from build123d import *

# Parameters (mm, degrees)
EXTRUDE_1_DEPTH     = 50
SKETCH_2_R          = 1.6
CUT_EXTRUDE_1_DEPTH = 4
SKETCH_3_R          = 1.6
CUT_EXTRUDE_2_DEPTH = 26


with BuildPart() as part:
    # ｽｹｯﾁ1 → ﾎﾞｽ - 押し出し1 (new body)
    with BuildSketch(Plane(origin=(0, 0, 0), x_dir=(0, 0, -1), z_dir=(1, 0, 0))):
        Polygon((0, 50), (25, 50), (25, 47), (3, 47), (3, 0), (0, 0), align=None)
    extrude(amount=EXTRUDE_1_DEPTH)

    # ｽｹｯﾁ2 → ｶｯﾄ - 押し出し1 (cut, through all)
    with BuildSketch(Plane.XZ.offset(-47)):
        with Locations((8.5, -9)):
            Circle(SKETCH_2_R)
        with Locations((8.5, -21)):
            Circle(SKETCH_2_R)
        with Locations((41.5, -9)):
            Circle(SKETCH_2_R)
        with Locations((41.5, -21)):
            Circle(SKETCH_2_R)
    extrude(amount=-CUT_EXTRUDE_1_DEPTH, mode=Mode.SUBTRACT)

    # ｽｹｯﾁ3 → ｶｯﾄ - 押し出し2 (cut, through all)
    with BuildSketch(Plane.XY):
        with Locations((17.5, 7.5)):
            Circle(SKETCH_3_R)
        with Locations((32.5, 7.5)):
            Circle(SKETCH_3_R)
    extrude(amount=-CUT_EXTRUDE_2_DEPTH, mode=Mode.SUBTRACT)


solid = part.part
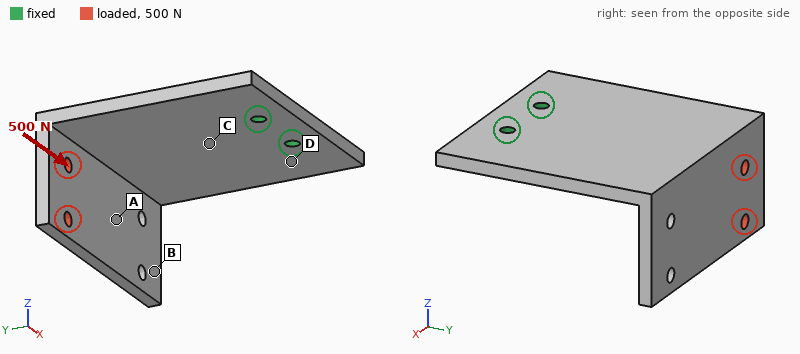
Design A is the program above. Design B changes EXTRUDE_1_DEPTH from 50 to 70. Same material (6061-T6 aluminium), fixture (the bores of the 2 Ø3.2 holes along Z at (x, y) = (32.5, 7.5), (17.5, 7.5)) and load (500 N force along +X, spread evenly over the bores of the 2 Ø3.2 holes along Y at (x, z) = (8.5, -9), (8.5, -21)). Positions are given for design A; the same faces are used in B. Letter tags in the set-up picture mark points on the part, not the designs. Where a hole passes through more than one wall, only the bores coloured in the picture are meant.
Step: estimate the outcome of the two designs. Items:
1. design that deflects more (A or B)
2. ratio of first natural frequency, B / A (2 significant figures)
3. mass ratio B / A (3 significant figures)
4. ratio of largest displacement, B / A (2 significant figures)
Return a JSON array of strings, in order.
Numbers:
["B", "0.85", "1.41", "1.2"]
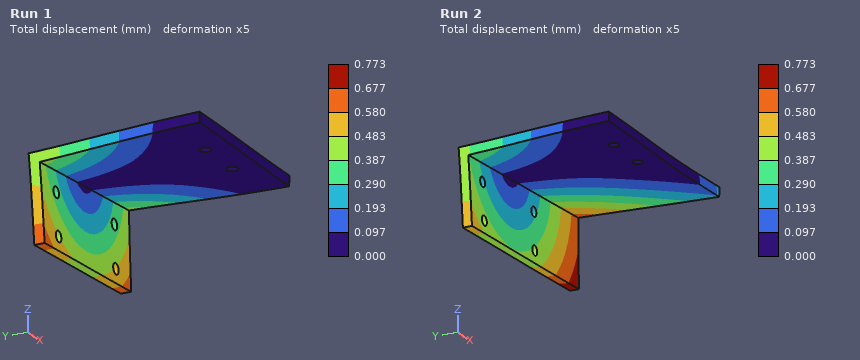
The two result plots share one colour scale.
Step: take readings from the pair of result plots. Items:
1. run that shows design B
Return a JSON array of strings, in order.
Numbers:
["Run 2"]
